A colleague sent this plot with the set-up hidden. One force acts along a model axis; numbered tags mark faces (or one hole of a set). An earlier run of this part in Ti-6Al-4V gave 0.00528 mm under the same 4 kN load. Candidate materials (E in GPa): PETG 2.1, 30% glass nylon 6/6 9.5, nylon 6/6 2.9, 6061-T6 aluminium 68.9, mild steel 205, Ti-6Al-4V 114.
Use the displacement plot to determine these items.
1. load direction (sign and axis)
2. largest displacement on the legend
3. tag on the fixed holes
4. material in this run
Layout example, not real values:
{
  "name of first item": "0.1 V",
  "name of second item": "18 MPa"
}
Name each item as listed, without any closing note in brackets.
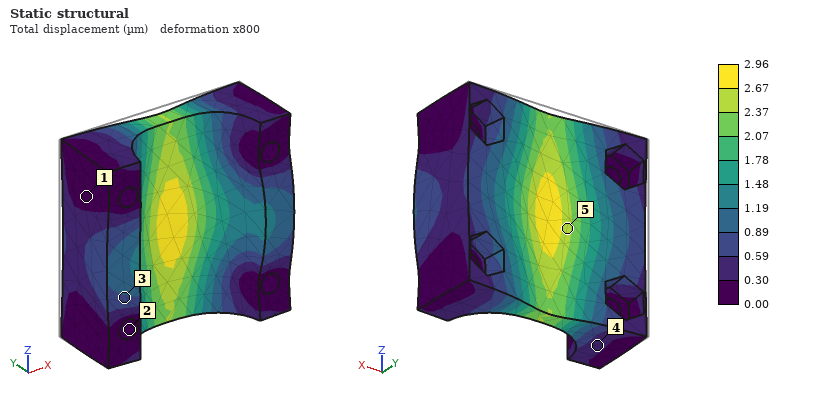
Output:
{
  "load direction": "-Y",
  "largest displacement on the legend": "2.96 µm",
  "tag on the fixed holes": "2",
  "material in this run": "mild steel"
}
